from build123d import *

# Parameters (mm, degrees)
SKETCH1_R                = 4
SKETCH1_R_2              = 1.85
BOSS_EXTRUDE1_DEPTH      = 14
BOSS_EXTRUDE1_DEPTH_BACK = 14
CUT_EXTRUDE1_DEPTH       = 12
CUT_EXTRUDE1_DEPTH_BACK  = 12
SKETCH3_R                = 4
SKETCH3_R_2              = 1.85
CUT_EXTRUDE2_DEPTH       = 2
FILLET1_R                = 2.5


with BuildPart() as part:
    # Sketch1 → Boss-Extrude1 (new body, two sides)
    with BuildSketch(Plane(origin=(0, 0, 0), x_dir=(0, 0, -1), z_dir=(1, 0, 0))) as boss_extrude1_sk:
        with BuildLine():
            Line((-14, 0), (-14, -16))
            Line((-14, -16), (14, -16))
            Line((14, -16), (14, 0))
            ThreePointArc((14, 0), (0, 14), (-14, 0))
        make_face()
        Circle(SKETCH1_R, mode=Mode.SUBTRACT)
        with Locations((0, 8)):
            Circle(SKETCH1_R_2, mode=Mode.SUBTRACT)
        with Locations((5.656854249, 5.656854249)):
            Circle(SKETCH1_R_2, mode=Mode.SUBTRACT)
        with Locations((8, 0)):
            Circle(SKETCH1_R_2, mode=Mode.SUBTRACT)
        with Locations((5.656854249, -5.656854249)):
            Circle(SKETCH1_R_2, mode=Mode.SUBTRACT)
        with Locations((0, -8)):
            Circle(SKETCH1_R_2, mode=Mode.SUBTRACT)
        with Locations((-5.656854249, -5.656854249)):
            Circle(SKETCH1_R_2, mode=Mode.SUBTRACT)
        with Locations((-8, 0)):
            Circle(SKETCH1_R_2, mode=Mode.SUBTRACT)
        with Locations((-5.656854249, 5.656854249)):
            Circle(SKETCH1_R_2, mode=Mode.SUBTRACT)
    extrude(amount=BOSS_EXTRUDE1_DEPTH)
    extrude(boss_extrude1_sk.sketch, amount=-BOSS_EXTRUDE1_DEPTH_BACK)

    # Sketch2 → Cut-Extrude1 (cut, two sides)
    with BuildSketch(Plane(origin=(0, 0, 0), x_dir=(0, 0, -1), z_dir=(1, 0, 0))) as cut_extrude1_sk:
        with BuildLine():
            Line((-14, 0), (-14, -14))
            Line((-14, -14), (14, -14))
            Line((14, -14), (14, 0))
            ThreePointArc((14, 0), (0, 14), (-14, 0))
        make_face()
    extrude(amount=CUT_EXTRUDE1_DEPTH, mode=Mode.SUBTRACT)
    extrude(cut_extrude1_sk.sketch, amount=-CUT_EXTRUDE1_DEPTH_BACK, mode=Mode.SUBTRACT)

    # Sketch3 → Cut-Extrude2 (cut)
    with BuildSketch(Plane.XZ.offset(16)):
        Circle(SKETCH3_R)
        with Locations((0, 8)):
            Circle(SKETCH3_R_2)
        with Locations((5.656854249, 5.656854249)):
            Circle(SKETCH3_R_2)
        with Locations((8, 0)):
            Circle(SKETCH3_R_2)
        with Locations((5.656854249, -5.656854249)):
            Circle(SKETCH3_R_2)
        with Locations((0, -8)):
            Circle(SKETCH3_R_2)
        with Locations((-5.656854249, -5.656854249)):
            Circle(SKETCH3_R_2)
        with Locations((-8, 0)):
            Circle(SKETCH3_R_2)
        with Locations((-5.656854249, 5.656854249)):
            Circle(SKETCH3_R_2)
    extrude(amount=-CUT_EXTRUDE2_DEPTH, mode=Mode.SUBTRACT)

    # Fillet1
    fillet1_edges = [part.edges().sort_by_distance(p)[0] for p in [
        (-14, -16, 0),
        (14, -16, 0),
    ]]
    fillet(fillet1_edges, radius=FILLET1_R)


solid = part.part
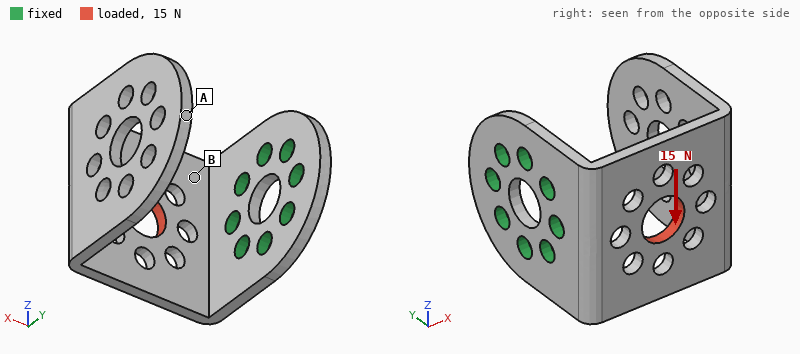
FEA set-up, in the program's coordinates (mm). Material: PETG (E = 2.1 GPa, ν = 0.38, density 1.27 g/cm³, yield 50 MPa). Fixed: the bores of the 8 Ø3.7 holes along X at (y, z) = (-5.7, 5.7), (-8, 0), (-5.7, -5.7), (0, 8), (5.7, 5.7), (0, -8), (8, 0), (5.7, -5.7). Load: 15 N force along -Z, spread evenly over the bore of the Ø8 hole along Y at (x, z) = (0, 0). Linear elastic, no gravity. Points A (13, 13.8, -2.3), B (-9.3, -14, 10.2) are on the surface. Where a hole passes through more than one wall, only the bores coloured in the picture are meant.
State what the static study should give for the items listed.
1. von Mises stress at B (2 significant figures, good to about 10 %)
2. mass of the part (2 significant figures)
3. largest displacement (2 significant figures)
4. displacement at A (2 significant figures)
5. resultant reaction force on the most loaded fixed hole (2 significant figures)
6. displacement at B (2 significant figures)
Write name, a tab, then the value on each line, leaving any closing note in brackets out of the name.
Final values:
von Mises stress at B	2.5 MPa
mass of the part	4.4 g
largest displacement	0.50 mm
displacement at A	0.50 mm
resultant reaction force on the most loaded fixed hole	13 N
displacement at B	0.10 mm
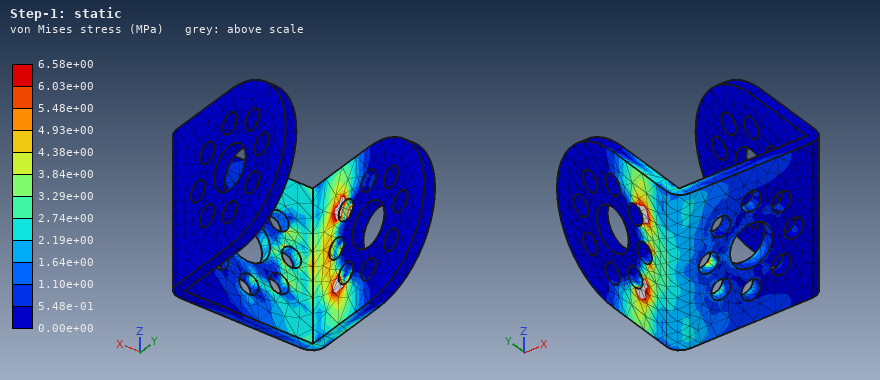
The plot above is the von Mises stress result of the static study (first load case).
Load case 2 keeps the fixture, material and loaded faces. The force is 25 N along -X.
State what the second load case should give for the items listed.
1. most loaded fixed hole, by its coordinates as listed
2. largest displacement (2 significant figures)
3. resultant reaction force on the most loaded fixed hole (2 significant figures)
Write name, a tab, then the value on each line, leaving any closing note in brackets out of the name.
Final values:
most loaded fixed hole, by its coordinates as listed	(-8, 0)
largest displacement	0.50 mm
resultant reaction force on the most loaded fixed hole	20 N
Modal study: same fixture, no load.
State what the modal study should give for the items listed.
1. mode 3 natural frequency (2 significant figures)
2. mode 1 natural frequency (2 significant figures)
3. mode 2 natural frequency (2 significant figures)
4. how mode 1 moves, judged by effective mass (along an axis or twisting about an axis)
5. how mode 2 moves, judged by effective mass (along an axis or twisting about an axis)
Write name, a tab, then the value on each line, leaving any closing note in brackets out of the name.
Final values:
mode 3 natural frequency	480 Hz
mode 1 natural frequency	170 Hz
mode 2 natural frequency	280 Hz
how mode 1 moves, judged by effective mass	along Y
how mode 2 moves, judged by effective mass	along Z
